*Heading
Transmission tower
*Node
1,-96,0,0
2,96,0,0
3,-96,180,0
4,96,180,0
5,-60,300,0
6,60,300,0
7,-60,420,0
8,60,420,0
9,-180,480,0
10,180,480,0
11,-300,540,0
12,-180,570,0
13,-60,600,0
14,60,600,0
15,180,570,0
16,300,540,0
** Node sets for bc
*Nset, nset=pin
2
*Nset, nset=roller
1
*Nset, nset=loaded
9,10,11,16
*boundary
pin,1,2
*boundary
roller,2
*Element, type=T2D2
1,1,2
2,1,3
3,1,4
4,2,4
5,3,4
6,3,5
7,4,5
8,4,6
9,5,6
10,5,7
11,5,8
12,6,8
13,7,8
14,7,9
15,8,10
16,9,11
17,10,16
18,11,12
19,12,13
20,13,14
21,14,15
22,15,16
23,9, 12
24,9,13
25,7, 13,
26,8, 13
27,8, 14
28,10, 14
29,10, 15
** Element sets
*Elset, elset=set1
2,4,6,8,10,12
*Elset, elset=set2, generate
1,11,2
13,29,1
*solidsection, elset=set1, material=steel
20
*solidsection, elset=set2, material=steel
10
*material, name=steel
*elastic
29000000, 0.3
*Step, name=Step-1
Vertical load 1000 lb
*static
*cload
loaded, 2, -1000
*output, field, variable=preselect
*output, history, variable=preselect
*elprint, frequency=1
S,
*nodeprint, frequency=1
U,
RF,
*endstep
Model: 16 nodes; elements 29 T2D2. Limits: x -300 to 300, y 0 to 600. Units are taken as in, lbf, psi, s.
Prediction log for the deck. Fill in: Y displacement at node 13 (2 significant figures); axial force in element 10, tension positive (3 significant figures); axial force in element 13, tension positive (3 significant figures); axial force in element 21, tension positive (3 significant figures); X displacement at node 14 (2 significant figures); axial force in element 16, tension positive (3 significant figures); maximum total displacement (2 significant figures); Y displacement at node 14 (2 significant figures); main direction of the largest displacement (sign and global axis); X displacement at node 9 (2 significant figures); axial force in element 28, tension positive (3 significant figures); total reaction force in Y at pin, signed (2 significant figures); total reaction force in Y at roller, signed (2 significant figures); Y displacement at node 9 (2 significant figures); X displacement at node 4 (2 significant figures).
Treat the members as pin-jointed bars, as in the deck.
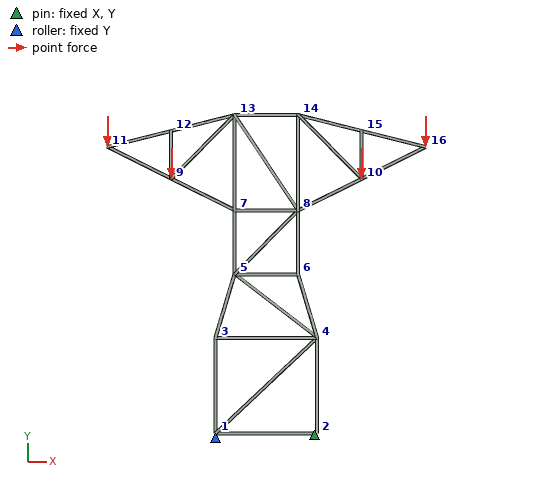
-0.0021 in
-2000 lbf
-2000 lbf
1370 lbf
9.6e-04 in
-1490 lbf
0.0079 in
-0.0023 in
-Y
0.0014 in
943 lbf
2000 lbf
2000 lbf
-0.0042 in
5.8e-04 in
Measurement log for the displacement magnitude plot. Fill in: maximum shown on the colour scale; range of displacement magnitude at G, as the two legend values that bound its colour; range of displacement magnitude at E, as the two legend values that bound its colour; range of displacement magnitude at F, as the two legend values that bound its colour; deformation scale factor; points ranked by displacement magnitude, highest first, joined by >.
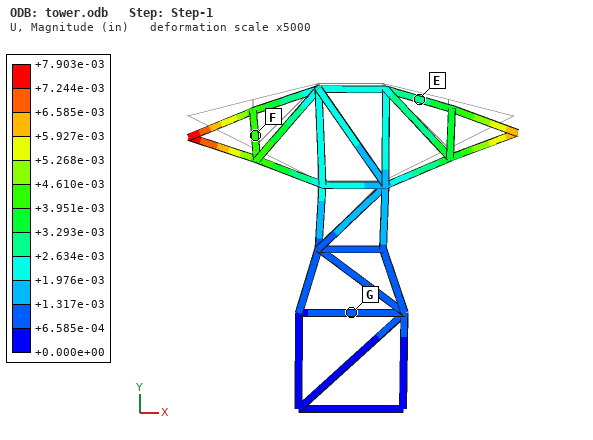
+7.903e-03 in
+6.585e-04 to +1.317e-03 in
+2.634e-03 to +3.293e-03 in
+3.951e-03 to +4.610e-03 in
5000
F > E > G
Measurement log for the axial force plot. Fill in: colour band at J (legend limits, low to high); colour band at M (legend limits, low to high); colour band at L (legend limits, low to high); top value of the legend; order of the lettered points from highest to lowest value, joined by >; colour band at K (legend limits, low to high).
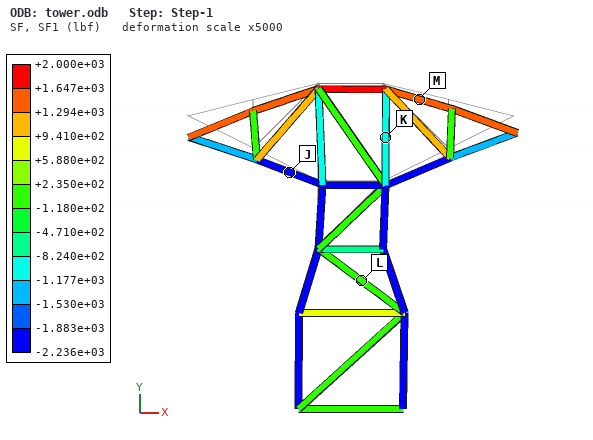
-2.236e+03 to -1.883e+03 lbf
+1.294e+03 to +1.647e+03 lbf
-1.180e+02 to +2.350e+02 lbf
+2.000e+03 lbf
M > L > K > J
-1.177e+03 to -8.240e+02 lbf
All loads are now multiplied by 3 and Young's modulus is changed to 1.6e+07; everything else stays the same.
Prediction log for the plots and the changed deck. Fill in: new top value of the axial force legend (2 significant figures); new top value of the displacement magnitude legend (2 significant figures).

6000 lbf
0.043 in
